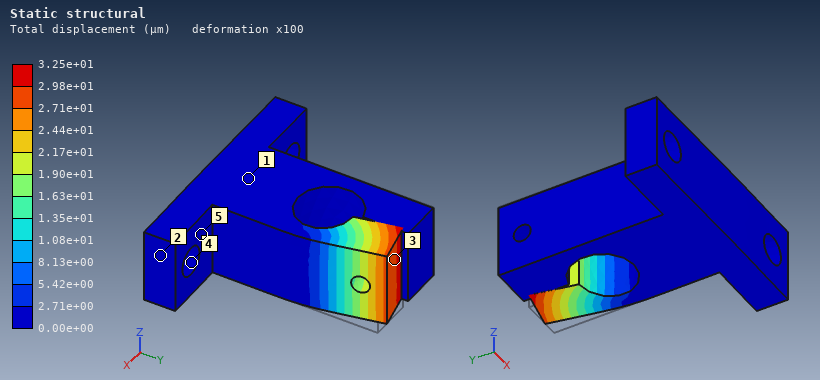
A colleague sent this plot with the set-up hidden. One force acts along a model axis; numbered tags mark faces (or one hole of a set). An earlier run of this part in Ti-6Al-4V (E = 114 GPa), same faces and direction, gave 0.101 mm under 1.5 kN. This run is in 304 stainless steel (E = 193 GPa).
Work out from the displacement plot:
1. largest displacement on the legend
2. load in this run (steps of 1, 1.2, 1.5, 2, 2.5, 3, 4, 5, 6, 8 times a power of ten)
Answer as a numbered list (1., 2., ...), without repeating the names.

1. 3.25e+01 µm
2. 800 N
